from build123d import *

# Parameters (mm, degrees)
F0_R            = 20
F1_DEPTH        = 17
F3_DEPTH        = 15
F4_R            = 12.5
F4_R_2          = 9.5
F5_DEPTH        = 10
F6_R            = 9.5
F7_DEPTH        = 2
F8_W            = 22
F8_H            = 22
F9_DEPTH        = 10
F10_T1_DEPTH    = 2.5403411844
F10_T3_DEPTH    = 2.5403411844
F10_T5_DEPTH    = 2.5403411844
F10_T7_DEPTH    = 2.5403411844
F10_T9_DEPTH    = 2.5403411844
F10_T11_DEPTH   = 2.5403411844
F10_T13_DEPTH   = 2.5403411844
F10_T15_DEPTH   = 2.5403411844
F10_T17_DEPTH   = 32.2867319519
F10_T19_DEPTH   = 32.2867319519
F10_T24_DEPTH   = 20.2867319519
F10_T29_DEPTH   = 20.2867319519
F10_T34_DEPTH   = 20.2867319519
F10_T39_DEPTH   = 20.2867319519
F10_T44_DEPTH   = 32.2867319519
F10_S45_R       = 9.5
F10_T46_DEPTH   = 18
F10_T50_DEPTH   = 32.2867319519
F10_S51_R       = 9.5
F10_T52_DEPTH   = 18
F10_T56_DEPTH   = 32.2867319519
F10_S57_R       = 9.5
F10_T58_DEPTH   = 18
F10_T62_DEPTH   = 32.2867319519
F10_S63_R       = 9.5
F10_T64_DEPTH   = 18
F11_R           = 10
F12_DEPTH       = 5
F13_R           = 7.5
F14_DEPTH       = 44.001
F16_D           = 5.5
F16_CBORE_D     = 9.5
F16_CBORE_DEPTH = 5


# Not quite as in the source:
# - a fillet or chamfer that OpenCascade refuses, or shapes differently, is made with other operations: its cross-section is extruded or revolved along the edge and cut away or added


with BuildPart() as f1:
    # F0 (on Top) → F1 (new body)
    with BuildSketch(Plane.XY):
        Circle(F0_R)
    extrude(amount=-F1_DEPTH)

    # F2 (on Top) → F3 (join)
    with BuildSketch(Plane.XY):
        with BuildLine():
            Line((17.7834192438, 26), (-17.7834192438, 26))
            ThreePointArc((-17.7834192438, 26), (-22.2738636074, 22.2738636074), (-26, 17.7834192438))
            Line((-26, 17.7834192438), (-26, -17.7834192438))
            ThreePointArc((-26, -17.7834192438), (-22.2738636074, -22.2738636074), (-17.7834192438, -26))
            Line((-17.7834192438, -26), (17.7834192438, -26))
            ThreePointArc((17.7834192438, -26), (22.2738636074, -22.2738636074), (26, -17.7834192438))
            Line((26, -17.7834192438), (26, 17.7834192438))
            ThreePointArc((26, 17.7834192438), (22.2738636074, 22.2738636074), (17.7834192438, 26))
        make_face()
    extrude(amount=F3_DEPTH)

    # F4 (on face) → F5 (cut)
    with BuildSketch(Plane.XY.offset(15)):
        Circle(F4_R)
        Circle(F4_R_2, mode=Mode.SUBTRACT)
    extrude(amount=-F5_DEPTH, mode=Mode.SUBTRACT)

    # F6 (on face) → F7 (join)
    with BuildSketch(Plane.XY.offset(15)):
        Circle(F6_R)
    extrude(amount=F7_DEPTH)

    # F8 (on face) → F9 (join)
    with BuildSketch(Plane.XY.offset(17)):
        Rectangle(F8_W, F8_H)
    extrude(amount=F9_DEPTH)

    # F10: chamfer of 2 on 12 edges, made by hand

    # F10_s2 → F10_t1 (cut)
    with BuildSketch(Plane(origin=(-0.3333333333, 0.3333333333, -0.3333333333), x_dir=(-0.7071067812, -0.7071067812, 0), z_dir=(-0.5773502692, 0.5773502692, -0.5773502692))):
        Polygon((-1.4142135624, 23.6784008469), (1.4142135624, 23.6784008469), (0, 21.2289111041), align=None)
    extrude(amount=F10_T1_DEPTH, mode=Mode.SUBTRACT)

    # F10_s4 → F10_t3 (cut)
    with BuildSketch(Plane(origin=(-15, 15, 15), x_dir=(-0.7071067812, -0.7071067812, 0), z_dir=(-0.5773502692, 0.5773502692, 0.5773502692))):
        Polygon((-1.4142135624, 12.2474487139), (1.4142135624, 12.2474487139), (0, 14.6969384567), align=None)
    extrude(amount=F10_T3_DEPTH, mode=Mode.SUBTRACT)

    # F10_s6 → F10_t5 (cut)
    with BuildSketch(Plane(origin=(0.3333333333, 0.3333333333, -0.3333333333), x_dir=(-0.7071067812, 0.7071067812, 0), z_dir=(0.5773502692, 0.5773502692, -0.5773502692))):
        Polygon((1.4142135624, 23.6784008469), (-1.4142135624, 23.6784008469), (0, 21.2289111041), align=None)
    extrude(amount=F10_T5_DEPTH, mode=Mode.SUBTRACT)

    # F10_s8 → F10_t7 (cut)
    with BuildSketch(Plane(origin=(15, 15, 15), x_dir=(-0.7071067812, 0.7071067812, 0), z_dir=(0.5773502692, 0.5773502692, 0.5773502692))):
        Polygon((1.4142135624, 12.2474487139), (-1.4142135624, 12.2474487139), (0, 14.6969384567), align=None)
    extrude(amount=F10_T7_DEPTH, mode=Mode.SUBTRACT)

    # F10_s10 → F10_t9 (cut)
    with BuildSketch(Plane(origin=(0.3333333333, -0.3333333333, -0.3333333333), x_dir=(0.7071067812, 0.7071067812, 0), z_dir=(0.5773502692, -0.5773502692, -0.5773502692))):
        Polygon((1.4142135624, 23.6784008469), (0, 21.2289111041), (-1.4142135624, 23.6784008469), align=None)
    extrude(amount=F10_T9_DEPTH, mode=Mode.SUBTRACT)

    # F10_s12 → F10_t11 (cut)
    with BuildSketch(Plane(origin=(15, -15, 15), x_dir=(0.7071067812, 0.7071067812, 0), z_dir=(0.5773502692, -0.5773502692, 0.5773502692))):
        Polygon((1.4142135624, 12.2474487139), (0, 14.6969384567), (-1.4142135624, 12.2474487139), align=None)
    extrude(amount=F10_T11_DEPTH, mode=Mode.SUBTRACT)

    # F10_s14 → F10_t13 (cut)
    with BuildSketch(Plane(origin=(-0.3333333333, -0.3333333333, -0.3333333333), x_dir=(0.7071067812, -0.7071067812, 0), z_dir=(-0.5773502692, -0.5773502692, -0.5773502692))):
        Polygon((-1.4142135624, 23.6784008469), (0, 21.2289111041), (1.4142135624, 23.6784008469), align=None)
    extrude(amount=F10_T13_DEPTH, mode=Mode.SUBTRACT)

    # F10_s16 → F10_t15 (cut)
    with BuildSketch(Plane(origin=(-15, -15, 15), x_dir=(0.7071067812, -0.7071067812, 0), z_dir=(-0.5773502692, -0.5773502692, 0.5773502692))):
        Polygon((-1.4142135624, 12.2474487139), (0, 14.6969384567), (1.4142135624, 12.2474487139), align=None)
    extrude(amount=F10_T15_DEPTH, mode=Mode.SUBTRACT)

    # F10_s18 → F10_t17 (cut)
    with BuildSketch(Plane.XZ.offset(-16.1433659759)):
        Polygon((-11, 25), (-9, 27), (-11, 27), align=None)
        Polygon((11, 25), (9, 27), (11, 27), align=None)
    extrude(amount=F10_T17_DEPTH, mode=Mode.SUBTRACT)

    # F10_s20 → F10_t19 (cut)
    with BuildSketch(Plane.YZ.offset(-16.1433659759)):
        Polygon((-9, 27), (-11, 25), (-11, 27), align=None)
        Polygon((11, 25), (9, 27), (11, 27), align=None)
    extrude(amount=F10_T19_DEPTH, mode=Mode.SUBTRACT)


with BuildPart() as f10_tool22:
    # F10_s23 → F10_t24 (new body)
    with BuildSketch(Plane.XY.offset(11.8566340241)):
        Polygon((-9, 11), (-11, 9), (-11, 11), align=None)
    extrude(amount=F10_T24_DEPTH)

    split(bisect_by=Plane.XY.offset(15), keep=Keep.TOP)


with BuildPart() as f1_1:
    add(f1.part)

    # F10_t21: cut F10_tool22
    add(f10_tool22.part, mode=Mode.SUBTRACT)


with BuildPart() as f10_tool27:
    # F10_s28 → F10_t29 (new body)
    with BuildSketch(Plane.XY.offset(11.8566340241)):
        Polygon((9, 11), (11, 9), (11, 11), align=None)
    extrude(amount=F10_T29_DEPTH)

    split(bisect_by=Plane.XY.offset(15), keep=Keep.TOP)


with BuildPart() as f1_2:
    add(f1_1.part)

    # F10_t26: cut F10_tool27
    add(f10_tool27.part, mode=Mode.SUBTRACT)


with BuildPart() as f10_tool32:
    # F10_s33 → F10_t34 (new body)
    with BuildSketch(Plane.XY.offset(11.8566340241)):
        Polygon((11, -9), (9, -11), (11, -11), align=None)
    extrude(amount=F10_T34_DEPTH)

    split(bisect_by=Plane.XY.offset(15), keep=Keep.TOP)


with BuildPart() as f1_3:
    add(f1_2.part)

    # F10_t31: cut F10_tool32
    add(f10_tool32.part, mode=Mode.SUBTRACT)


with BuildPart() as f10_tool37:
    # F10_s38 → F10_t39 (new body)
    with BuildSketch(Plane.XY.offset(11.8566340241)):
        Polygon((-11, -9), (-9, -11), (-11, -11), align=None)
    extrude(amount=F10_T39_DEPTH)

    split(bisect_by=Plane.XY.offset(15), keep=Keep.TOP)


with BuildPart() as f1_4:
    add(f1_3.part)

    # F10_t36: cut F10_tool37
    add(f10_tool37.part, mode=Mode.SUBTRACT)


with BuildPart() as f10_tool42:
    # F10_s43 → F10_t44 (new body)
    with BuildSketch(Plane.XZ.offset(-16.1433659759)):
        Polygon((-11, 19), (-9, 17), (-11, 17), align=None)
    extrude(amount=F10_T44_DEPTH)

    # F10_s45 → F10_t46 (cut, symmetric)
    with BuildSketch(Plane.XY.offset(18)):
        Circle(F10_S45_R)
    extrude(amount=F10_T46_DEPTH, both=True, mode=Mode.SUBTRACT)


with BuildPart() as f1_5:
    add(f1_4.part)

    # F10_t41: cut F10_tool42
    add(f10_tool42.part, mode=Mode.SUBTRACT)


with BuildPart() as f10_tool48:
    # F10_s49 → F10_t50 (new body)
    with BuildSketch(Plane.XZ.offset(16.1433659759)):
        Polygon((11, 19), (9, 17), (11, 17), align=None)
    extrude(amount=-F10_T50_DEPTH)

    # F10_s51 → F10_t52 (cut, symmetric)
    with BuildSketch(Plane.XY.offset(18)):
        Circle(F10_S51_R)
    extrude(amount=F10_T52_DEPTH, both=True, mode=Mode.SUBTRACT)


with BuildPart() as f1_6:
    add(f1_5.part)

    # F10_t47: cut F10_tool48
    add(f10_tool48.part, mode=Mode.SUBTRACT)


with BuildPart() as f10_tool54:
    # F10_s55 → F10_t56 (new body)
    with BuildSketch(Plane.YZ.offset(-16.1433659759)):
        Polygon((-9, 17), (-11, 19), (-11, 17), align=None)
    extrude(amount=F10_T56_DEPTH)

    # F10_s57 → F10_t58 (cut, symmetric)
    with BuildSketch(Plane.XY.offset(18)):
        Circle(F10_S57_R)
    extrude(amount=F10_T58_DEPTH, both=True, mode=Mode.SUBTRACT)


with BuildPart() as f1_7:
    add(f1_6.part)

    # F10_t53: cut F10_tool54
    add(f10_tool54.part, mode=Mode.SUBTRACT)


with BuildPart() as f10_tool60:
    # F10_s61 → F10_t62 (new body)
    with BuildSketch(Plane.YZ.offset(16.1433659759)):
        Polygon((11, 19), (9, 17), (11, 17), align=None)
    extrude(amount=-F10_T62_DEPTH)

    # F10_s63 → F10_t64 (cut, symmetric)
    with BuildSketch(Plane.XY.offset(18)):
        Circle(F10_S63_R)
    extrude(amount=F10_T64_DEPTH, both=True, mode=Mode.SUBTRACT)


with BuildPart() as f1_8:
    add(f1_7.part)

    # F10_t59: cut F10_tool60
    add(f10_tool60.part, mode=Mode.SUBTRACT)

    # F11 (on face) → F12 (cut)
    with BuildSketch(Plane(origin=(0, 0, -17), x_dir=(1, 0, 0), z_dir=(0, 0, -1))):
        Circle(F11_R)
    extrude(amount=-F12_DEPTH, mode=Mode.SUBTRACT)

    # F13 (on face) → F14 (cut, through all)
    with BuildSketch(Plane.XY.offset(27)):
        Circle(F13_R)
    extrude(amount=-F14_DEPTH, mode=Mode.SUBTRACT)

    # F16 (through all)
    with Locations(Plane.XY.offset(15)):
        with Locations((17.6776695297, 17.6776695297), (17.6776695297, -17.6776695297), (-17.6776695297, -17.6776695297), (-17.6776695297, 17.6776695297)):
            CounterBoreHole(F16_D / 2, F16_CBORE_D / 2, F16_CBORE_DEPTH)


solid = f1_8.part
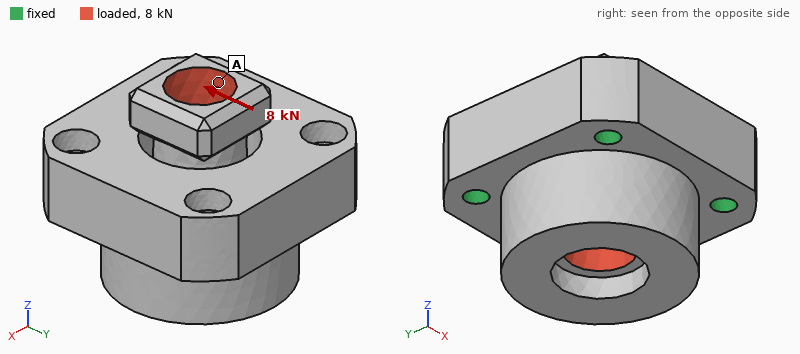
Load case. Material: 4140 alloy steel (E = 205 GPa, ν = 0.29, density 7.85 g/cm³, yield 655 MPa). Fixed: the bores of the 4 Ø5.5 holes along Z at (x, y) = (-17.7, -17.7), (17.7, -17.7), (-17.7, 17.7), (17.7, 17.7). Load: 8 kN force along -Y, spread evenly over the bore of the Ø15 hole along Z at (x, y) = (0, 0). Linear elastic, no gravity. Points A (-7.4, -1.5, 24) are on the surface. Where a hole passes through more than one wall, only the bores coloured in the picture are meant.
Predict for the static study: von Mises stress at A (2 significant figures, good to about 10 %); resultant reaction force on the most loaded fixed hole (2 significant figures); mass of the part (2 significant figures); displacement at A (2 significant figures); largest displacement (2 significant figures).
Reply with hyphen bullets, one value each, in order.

- 18 MPa
- 2.1 kN
- 410 g
- 23 µm
- 27 µm
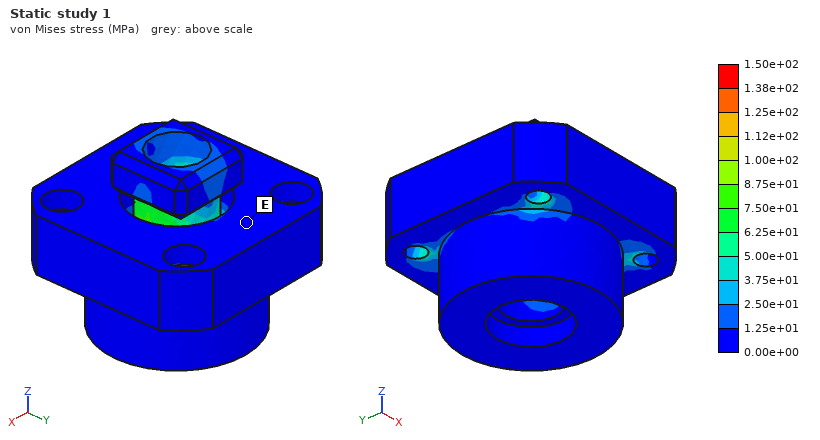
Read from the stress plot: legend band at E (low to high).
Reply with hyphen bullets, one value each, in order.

- 0.00e+00 to 1.25e+01 MPa
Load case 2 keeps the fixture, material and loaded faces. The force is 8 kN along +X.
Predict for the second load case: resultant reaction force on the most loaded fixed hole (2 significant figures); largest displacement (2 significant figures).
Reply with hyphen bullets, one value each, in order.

- 2.1 kN
- 27 µm
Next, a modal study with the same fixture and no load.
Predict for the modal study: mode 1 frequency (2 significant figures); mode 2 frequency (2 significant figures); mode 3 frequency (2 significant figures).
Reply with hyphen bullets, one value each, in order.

- 12 kHz
- 12 kHz
- 20 kHz
